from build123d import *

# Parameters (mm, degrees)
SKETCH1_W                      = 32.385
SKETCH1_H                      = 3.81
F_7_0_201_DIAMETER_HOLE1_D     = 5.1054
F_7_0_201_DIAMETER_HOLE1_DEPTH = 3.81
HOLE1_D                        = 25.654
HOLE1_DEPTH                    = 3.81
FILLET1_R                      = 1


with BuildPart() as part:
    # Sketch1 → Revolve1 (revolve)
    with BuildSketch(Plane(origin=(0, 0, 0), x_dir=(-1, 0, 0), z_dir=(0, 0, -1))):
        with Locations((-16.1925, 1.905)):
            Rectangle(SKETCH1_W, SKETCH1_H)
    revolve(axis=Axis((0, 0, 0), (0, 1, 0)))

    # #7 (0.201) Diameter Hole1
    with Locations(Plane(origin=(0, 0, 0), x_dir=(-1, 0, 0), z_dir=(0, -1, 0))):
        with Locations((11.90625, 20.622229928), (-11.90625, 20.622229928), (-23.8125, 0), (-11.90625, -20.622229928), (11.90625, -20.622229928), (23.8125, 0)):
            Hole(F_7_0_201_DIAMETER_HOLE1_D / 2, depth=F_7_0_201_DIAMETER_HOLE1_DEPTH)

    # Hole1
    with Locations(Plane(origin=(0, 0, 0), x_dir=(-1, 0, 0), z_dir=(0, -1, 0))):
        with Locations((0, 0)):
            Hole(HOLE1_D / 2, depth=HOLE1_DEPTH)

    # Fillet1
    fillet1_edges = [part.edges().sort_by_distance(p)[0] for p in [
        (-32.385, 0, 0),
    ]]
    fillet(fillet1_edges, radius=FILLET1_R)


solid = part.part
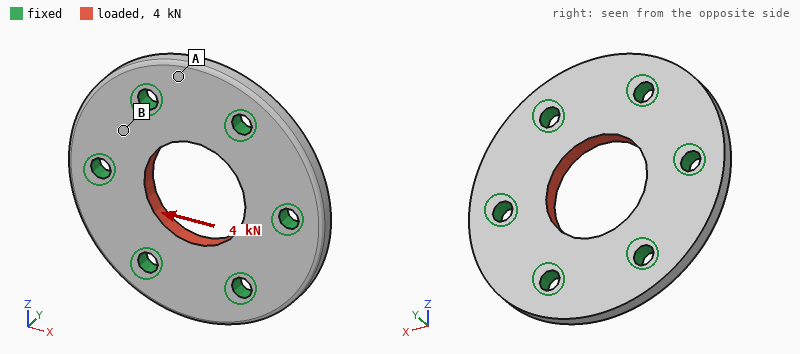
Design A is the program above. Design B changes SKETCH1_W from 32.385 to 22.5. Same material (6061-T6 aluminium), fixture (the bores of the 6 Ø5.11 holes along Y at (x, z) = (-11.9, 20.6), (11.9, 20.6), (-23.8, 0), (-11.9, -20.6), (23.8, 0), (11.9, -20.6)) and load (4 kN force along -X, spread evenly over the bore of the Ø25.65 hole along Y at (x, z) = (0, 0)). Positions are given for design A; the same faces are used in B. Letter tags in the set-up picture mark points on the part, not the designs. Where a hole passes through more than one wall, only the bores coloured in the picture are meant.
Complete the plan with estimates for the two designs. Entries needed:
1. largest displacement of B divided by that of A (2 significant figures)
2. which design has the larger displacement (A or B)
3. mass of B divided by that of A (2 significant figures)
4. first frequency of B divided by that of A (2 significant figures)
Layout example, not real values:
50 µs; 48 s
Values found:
1.1; B; 0.65; 1.2
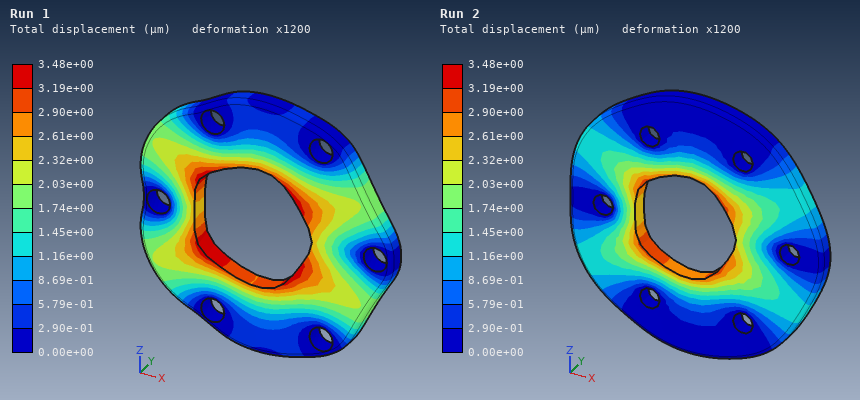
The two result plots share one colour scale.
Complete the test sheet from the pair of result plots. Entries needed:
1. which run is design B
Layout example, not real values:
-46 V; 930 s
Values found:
Run 1
